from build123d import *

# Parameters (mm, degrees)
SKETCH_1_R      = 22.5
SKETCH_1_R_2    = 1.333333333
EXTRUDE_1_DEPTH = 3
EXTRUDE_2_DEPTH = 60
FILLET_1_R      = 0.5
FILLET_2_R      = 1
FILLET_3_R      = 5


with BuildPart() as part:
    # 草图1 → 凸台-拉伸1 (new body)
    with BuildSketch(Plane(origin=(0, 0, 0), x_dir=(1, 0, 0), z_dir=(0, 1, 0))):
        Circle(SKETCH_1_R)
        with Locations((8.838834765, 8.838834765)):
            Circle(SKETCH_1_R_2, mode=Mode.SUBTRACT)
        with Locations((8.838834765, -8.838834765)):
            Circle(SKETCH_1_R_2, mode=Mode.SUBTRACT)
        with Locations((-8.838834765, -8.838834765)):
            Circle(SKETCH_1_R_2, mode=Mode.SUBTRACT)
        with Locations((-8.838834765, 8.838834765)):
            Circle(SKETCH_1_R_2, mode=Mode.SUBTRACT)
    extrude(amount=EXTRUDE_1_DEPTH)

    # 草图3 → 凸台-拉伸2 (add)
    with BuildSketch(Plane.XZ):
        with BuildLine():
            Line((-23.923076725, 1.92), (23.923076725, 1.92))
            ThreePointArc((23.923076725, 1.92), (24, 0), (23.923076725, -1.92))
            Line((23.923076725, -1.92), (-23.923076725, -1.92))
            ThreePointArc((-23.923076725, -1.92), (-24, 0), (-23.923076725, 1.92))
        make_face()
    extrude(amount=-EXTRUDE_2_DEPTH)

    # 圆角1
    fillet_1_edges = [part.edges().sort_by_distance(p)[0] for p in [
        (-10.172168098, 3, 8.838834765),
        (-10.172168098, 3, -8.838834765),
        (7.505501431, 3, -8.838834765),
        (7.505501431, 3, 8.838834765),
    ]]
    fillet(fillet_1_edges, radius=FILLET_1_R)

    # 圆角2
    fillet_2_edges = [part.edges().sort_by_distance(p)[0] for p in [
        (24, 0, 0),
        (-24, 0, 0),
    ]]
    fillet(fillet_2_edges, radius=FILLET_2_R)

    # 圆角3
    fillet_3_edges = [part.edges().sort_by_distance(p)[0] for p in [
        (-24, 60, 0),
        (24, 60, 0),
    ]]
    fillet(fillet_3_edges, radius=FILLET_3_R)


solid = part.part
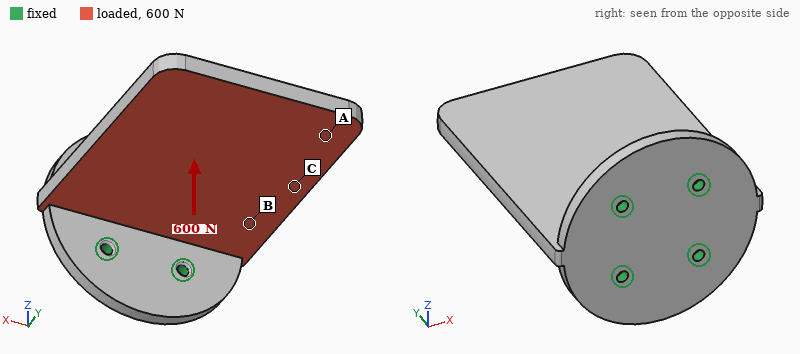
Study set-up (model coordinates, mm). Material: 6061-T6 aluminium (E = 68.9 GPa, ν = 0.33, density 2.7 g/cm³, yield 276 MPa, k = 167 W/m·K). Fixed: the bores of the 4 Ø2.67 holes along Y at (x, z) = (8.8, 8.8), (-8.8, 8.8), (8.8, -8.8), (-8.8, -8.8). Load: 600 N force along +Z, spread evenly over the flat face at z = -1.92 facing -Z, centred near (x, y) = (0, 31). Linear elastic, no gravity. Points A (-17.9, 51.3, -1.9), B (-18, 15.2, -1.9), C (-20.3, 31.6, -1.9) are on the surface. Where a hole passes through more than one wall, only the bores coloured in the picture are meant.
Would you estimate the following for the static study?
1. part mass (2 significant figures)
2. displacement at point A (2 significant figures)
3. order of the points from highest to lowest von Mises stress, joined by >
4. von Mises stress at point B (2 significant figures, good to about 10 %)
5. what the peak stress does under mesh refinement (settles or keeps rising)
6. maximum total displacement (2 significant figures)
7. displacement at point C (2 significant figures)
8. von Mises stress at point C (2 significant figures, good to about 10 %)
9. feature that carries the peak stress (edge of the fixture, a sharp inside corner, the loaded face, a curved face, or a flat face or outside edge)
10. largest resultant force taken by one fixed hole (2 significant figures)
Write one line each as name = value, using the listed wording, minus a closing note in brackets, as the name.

part mass = 41 g
displacement at point A = 0.85 mm
order of the points from highest to lowest von Mises stress, joined by > = B > C > A
von Mises stress at point B = 83 MPa
what the peak stress does under mesh refinement = keeps rising
maximum total displacement = 1.1 mm
displacement at point C = 0.40 mm
von Mises stress at point C = 37 MPa
feature that carries the peak stress = edge of the fixture
largest resultant force taken by one fixed hole = 630 N
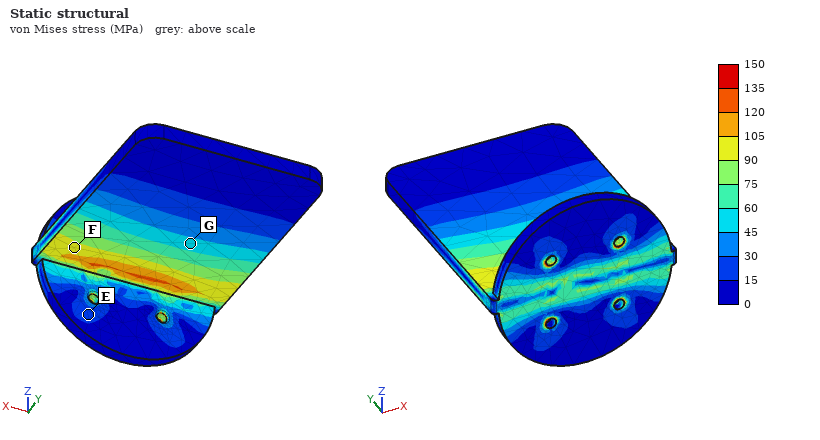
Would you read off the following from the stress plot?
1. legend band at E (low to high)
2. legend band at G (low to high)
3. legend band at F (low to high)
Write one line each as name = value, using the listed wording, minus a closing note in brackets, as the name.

legend band at E = 15 to 30 MPa
legend band at G = 45 to 60 MPa
legend band at F = 90 to 105 MPa
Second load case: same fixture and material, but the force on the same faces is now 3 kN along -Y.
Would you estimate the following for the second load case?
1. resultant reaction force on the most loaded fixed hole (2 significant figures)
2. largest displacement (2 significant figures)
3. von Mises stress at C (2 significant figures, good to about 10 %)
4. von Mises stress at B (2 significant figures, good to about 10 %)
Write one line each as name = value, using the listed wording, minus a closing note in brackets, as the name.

resultant reaction force on the most loaded fixed hole = 970 N
largest displacement = 0.45 mm
von Mises stress at C = 31 MPa
von Mises stress at B = 45 MPa
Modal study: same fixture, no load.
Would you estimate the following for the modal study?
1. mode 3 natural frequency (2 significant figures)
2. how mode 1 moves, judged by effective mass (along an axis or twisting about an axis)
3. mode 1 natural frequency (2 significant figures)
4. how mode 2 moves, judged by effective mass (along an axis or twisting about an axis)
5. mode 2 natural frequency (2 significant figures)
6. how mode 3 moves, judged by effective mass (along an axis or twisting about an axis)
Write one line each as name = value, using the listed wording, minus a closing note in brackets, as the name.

mode 3 natural frequency = 2800 Hz
how mode 1 moves, judged by effective mass = along Z
mode 1 natural frequency = 890 Hz
how mode 2 moves, judged by effective mass = twisting about Y
mode 2 natural frequency = 2500 Hz
how mode 3 moves, judged by effective mass = along X
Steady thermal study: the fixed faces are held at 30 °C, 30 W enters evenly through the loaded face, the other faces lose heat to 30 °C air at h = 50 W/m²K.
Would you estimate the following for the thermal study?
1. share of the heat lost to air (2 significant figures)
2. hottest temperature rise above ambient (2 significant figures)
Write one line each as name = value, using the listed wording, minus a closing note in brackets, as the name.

share of the heat lost to air = 15 %
hottest temperature rise above ambient = 31 K
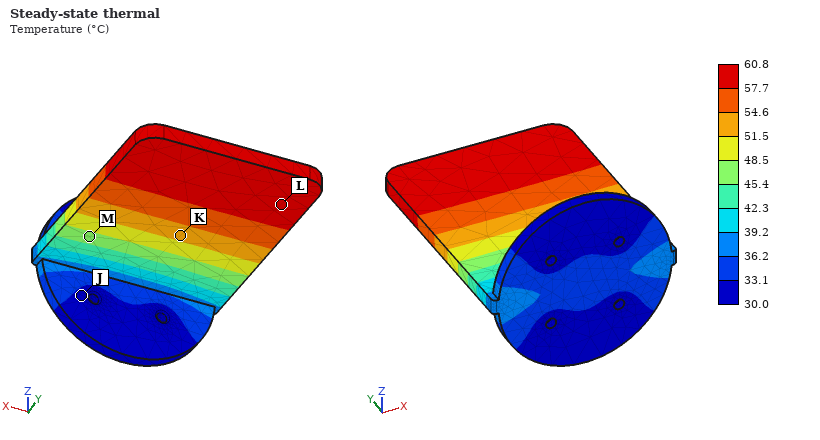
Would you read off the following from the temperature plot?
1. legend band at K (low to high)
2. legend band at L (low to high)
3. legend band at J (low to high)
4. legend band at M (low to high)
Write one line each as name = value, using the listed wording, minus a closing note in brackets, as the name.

legend band at K = 51.5 to 54.6 °C
legend band at L = 57.7 to 60.8 °C
legend band at J = 30.0 to 33.1 °C
legend band at M = 45.4 to 48.5 °C
